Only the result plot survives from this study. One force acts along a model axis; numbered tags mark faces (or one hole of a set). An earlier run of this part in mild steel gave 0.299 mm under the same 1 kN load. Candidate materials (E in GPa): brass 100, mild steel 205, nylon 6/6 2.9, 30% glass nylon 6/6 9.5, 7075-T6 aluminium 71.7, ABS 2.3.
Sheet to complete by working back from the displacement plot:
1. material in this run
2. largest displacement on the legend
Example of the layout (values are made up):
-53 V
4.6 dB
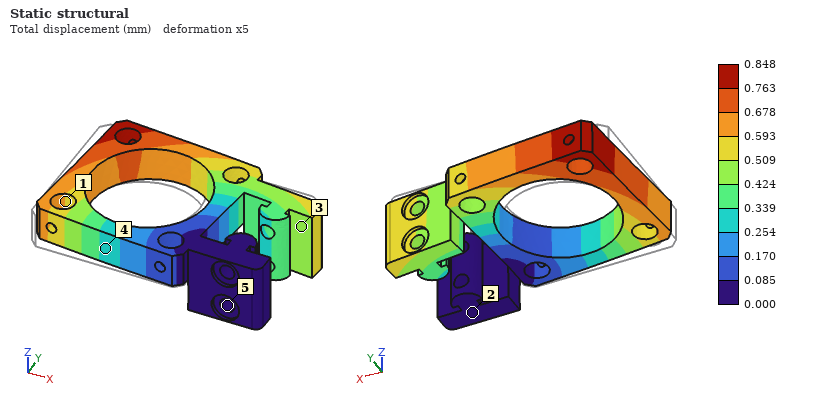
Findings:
7075-T6 aluminium
0.848 mm
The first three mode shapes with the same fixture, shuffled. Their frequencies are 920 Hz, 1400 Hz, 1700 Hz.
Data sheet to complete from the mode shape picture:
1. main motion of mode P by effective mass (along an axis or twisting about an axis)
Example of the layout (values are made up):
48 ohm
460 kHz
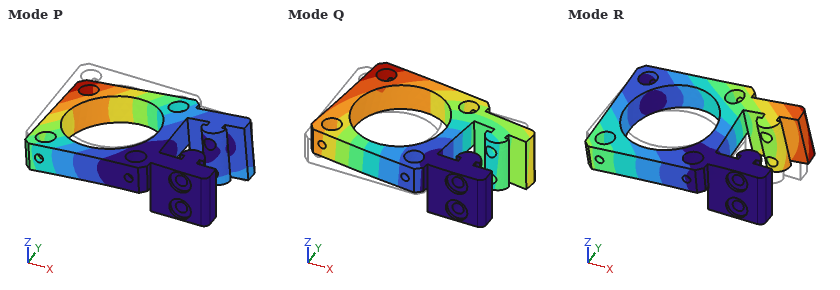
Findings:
along Z
